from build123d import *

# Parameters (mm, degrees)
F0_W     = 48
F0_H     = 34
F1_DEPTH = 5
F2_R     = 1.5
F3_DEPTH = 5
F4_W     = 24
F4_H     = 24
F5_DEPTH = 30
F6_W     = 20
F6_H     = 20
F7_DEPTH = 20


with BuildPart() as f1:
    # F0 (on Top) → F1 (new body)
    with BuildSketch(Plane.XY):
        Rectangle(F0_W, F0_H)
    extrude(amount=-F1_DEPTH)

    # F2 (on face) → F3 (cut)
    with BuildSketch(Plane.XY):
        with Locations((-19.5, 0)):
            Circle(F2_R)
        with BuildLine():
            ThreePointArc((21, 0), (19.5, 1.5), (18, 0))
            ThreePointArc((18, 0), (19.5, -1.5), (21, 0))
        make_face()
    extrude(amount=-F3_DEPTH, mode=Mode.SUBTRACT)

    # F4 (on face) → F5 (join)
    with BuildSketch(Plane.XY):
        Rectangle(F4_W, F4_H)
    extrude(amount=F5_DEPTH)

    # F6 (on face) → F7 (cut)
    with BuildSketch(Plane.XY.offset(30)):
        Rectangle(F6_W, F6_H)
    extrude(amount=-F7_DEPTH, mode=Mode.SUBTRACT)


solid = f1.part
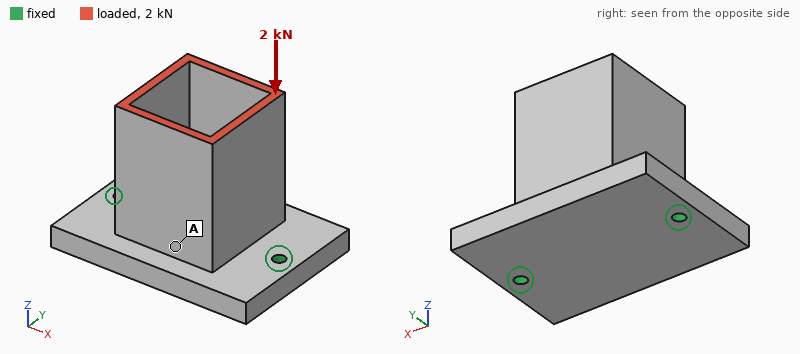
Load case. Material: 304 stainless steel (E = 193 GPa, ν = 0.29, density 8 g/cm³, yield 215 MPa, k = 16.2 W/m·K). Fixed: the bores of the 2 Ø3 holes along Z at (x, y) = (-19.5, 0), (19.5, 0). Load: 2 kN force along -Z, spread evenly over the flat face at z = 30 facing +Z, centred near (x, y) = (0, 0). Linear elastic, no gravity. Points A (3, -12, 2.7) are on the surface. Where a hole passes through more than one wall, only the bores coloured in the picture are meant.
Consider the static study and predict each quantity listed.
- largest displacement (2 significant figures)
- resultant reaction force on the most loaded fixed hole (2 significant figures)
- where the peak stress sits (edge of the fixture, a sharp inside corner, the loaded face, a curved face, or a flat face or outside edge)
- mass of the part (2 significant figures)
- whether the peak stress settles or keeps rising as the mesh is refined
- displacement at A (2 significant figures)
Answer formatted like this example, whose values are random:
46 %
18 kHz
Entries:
6.3 µm
1.1 kN
edge of the fixture
140 g
keeps rising
5.1 µm
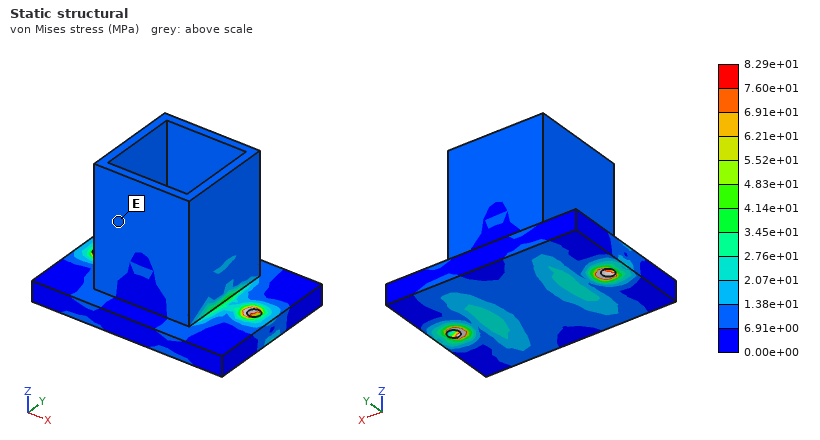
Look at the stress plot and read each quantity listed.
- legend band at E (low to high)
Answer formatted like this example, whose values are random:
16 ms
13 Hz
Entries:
6.91e+00 to 1.38e+01 MPa
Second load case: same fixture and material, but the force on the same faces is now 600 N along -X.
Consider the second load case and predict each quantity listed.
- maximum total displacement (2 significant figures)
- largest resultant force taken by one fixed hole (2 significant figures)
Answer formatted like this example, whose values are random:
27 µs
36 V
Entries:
19 µm
650 N
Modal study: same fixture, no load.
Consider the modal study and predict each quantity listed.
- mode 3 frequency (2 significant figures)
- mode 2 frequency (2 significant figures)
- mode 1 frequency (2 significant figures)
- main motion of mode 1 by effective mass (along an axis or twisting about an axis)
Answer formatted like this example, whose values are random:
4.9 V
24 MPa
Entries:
9300 Hz
9100 Hz
3500 Hz
along Y
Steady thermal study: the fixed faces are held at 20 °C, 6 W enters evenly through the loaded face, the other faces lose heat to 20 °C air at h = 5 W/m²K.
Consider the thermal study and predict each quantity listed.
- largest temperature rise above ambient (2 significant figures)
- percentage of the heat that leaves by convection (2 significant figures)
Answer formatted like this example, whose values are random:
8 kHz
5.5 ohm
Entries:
64 K
19 %
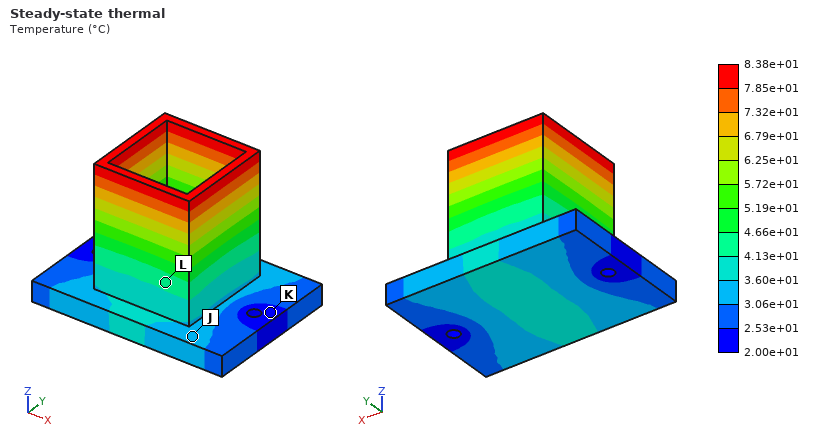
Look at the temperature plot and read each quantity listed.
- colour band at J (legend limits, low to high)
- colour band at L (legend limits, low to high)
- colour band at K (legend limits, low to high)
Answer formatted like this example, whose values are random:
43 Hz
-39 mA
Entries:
3.06e+01 to 3.60e+01 °C
4.13e+01 to 4.66e+01 °C
2.00e+01 to 2.53e+01 °C
